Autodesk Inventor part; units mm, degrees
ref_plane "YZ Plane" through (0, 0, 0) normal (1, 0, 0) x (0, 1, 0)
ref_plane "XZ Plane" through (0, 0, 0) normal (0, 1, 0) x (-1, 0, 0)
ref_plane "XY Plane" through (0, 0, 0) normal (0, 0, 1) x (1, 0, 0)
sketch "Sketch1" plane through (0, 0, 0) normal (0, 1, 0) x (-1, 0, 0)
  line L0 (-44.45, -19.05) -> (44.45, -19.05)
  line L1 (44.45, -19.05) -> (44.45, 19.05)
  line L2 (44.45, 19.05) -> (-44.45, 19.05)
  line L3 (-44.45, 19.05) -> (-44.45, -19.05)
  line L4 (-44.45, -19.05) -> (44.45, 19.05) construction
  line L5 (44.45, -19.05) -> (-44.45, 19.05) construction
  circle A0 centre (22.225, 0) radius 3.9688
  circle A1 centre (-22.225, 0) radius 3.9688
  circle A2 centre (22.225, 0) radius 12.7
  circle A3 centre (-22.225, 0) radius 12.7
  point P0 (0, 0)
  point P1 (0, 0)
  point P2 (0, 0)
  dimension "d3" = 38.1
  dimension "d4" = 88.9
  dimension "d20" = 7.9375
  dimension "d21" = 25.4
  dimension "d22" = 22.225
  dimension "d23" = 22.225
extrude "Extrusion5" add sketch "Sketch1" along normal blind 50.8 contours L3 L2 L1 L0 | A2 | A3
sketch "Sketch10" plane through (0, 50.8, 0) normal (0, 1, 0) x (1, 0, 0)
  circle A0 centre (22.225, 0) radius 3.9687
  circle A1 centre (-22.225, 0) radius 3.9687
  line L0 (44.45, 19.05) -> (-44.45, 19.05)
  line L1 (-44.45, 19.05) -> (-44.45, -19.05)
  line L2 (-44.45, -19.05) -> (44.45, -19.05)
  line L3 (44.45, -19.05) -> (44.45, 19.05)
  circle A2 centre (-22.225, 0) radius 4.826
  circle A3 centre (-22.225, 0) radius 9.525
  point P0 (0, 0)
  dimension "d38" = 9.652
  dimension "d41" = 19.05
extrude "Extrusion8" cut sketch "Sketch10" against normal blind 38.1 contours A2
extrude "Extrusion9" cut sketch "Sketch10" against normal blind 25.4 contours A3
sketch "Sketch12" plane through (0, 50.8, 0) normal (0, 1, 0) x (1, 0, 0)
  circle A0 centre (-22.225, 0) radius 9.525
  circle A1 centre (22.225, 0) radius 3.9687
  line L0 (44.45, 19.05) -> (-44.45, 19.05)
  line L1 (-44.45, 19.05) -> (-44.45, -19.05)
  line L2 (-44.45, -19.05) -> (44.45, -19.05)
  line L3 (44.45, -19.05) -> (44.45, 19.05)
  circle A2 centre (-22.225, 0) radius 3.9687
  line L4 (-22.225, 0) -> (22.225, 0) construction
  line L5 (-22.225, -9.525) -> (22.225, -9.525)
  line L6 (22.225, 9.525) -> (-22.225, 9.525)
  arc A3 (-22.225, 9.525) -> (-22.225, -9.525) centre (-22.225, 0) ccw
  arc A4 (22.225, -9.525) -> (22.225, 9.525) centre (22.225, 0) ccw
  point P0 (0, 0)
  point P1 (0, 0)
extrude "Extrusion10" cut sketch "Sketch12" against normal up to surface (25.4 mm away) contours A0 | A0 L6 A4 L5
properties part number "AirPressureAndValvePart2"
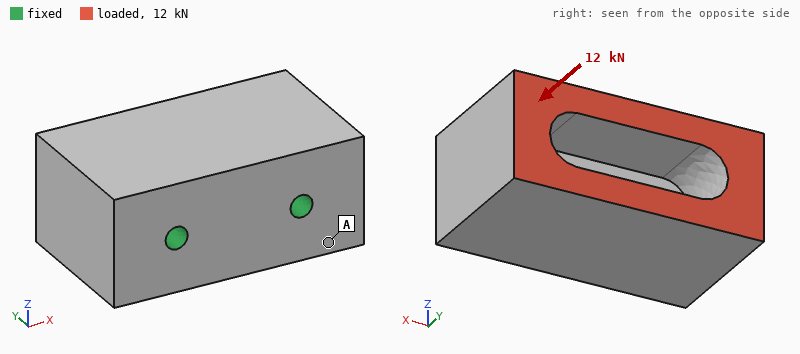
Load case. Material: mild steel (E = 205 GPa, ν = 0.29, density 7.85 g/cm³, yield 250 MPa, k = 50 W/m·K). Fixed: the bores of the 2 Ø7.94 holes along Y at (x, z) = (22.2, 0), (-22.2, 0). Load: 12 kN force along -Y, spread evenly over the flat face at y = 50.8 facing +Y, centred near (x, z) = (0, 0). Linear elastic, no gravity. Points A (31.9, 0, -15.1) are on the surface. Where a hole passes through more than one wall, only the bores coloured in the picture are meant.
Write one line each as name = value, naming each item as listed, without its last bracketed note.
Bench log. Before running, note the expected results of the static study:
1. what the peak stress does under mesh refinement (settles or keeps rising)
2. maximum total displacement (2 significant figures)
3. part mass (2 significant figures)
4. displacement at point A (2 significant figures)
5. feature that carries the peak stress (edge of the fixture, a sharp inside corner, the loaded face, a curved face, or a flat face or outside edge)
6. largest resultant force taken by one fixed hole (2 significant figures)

what the peak stress does under mesh refinement = keeps rising
maximum total displacement = 2.9 µm
part mass = 1.1 kg
displacement at point A = 0.87 µm
feature that carries the peak stress = edge of the fixture
largest resultant force taken by one fixed hole = 6.1 kN
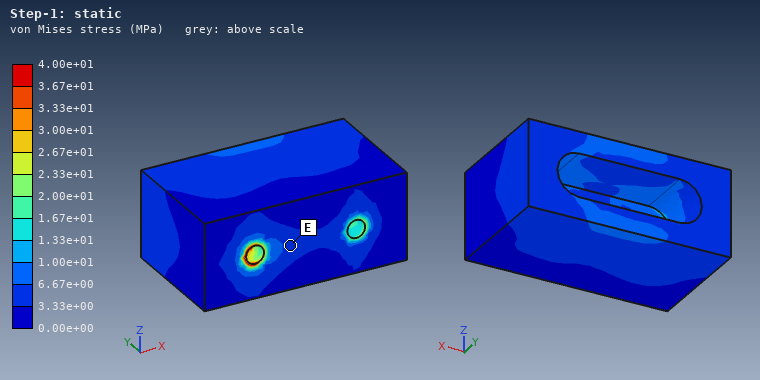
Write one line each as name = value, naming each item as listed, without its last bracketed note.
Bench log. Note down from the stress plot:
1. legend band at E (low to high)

legend band at E = 3.33e+00 to 6.67e+00 MPa
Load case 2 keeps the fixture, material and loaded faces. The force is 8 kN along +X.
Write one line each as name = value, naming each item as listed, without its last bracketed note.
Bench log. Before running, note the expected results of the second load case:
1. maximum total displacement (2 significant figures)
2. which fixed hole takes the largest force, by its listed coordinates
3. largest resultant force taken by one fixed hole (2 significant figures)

maximum total displacement = 7.5 µm
which fixed hole takes the largest force, by its listed coordinates = (22.2, 0)
largest resultant force taken by one fixed hole = 8.1 kN
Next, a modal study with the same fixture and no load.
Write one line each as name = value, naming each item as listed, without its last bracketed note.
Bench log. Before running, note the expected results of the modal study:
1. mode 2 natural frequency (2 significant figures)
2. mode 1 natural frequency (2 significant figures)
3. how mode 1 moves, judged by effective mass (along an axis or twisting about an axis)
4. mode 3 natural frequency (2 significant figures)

mode 2 natural frequency = 9800 Hz
mode 1 natural frequency = 5700 Hz
how mode 1 moves, judged by effective mass = along Z
mode 3 natural frequency = 10 kHz
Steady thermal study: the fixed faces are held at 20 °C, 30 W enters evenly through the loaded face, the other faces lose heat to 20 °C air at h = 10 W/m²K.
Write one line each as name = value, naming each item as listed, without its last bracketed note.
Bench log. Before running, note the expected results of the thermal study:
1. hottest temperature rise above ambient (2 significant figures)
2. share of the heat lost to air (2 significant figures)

hottest temperature rise above ambient = 13 K
share of the heat lost to air = 4.1 %
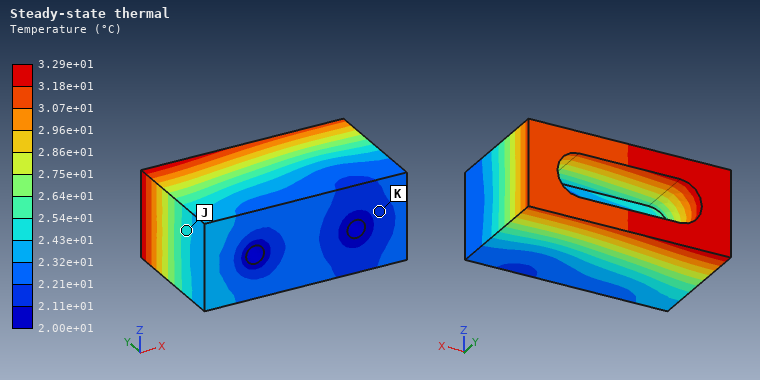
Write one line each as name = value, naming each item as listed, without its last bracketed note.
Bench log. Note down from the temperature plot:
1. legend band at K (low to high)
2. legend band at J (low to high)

legend band at K = 2.11e+01 to 2.21e+01 °C
legend band at J = 2.43e+01 to 2.54e+01 °C
